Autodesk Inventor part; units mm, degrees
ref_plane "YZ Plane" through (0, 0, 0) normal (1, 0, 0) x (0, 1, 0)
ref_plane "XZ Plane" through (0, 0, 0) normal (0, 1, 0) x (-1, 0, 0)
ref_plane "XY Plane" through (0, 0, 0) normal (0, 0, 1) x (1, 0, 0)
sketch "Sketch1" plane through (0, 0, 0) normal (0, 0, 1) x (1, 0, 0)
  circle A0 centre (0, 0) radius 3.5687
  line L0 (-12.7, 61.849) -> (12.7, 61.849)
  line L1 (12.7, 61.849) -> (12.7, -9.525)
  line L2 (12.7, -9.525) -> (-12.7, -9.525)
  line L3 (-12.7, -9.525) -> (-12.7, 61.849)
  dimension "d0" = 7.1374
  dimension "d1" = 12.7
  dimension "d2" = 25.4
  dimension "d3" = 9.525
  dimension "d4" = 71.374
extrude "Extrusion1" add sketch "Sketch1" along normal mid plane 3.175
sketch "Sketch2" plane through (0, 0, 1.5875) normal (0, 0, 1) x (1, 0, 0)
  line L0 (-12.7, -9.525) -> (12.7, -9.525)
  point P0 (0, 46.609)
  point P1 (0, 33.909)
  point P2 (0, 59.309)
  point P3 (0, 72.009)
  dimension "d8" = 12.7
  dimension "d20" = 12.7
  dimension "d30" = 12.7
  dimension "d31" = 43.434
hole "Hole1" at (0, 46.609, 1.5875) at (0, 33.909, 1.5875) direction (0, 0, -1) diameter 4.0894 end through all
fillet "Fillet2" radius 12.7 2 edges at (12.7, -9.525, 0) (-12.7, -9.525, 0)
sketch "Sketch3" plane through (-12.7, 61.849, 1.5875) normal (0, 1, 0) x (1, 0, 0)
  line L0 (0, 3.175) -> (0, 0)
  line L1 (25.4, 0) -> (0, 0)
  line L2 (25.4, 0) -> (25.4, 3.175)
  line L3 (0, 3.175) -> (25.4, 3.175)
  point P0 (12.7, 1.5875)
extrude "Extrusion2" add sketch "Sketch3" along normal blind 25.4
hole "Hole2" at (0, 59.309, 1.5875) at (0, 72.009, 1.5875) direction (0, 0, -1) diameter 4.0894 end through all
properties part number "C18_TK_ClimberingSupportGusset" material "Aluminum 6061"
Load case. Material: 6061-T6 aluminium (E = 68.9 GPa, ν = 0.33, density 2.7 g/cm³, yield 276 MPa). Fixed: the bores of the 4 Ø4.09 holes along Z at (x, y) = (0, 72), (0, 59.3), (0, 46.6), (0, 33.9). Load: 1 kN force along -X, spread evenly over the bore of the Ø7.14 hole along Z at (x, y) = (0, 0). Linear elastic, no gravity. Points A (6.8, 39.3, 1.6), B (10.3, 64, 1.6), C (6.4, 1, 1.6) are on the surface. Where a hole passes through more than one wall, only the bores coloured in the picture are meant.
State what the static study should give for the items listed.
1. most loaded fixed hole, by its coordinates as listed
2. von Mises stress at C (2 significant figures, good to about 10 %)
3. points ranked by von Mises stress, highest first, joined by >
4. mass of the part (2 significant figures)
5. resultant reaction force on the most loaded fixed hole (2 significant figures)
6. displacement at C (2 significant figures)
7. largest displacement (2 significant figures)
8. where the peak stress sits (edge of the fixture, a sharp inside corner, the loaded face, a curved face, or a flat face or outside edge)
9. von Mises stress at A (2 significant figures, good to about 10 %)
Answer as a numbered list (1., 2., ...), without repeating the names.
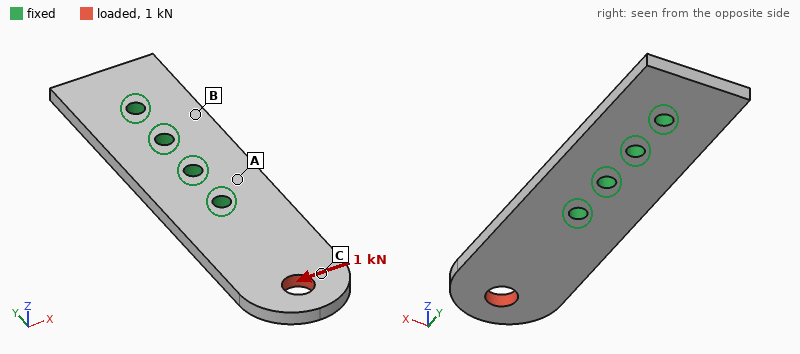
1. (0, 33.9)
2. 28 MPa
3. A > C > B
4. 20 g
5. 2.3 kN
6. 0.11 mm
7. 0.14 mm
8. edge of the fixture
9. 49 MPa
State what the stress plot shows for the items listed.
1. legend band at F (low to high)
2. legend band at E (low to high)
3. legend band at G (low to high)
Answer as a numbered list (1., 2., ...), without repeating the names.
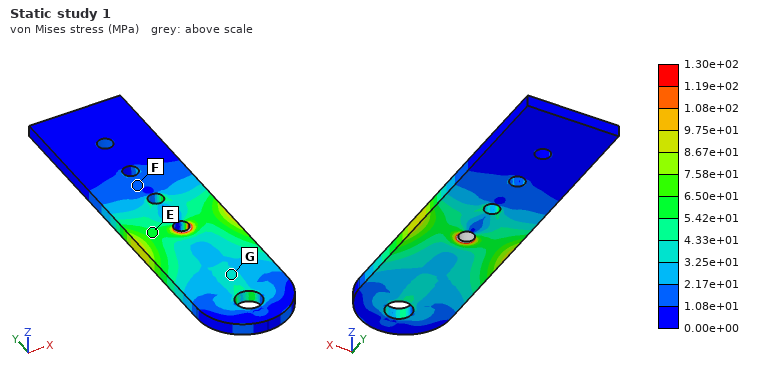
1. 1.08e+01 to 2.17e+01 MPa
2. 5.42e+01 to 6.50e+01 MPa
3. 3.25e+01 to 4.33e+01 MPa
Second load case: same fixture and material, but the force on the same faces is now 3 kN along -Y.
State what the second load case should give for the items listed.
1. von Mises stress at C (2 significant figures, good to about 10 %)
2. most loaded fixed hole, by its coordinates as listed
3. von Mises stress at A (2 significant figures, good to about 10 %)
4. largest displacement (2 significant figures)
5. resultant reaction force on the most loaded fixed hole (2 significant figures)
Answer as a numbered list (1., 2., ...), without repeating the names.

1. 42 MPa
2. (0, 33.9)
3. 19 MPa
4. 30 µm
5. 2.1 kN
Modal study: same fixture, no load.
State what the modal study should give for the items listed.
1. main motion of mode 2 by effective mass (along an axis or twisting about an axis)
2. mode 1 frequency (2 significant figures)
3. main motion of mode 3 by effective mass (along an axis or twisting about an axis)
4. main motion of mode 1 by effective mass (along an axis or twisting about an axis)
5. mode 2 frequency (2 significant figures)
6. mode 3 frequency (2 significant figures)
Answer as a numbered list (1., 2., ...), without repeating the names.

1. twisting about Y
2. 1600 Hz
3. along X
4. along Z
5. 4900 Hz
6. 7600 Hz
